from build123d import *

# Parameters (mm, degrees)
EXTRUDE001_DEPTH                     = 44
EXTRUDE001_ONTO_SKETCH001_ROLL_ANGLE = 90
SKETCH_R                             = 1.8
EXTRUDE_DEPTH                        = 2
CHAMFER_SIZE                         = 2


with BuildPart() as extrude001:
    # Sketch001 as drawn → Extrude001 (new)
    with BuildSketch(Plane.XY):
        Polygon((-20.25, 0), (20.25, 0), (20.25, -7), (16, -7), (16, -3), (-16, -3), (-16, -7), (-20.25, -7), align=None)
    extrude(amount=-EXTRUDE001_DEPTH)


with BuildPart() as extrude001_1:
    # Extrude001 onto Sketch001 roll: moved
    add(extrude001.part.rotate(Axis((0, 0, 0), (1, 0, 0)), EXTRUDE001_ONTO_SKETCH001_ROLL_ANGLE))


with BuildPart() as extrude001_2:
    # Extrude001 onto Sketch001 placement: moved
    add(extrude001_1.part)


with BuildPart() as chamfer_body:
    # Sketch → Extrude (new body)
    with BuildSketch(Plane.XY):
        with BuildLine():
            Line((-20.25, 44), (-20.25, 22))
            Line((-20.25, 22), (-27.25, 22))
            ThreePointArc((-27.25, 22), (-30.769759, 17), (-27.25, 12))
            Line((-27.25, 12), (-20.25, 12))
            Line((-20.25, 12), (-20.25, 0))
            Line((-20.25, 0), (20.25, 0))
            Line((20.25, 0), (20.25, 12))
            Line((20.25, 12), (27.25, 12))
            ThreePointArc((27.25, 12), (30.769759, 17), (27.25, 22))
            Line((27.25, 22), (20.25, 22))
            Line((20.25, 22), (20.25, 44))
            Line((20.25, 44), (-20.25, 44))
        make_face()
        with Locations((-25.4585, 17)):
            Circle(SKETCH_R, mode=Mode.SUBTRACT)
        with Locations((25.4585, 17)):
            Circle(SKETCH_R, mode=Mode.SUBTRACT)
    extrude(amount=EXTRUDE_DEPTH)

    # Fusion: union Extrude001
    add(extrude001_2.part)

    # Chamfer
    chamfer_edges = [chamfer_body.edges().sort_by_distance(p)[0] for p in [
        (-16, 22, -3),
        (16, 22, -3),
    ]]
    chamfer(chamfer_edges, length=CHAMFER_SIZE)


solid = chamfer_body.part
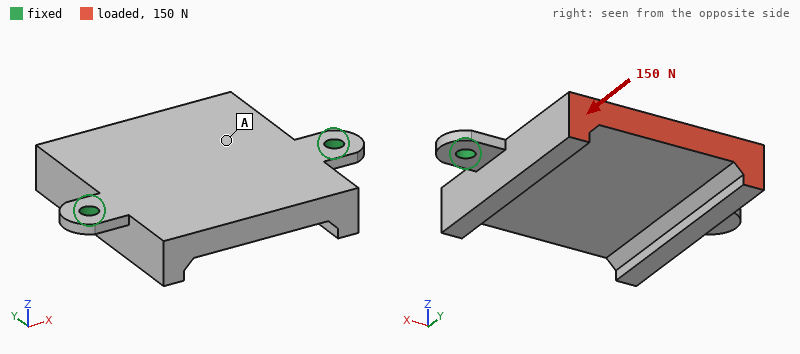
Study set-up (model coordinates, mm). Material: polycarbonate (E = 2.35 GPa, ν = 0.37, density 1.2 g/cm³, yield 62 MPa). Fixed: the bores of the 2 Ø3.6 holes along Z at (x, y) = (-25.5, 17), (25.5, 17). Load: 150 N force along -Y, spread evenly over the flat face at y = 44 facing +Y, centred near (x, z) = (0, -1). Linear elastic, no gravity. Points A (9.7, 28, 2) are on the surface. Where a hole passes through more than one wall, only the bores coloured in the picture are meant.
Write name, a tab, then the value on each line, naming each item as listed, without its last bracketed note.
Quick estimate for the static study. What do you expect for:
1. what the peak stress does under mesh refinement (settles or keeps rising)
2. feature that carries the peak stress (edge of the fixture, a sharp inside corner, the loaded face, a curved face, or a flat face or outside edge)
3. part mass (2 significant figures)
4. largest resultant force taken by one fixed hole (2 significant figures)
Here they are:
what the peak stress does under mesh refinement	keeps rising
feature that carries the peak stress	edge of the fixture
part mass	13 g
largest resultant force taken by one fixed hole	75 N
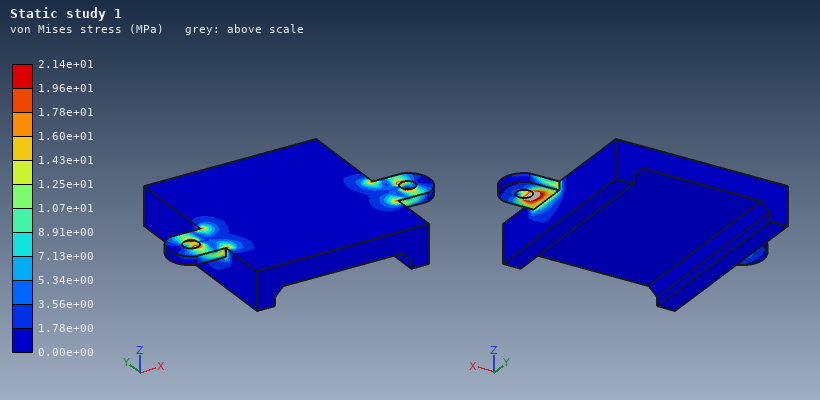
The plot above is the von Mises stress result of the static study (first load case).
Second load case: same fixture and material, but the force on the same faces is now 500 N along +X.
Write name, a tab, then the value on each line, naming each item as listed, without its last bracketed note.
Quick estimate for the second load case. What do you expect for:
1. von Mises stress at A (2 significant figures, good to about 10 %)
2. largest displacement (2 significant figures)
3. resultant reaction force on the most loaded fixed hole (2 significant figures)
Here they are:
von Mises stress at A	6.1 MPa
largest displacement	0.37 mm
resultant reaction force on the most loaded fixed hole	380 N
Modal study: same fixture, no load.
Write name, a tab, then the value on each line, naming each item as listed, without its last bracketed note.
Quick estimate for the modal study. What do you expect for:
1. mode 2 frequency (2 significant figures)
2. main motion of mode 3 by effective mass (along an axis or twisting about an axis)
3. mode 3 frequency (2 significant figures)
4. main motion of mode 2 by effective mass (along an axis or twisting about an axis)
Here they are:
mode 2 frequency	1400 Hz
main motion of mode 3 by effective mass	twisting about Y
mode 3 frequency	1900 Hz
main motion of mode 2 by effective mass	along Z
